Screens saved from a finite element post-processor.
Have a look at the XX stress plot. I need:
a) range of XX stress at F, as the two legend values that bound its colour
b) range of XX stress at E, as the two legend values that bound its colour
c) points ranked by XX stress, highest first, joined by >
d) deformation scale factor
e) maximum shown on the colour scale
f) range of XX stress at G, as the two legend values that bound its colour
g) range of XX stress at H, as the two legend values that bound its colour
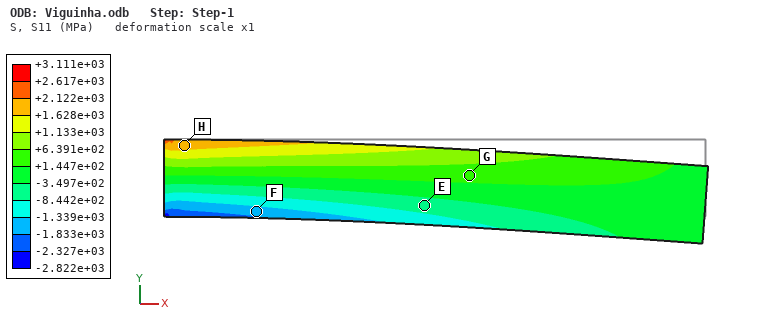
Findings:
-1.833e+03 to -1.339e+03 MPa
-8.442e+02 to -3.497e+02 MPa
H > G > E > F
1
+3.111e+03 MPa
+1.447e+02 to +6.391e+02 MPa
+1.628e+03 to +2.122e+03 MPa
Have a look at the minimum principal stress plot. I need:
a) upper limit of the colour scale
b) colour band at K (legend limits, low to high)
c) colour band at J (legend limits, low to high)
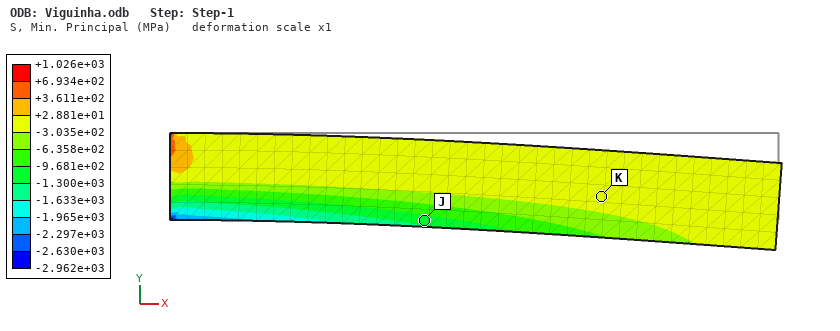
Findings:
+1.026e+03 MPa
-3.035e+02 to +2.881e+01 MPa
-1.300e+03 to -9.681e+02 MPa
